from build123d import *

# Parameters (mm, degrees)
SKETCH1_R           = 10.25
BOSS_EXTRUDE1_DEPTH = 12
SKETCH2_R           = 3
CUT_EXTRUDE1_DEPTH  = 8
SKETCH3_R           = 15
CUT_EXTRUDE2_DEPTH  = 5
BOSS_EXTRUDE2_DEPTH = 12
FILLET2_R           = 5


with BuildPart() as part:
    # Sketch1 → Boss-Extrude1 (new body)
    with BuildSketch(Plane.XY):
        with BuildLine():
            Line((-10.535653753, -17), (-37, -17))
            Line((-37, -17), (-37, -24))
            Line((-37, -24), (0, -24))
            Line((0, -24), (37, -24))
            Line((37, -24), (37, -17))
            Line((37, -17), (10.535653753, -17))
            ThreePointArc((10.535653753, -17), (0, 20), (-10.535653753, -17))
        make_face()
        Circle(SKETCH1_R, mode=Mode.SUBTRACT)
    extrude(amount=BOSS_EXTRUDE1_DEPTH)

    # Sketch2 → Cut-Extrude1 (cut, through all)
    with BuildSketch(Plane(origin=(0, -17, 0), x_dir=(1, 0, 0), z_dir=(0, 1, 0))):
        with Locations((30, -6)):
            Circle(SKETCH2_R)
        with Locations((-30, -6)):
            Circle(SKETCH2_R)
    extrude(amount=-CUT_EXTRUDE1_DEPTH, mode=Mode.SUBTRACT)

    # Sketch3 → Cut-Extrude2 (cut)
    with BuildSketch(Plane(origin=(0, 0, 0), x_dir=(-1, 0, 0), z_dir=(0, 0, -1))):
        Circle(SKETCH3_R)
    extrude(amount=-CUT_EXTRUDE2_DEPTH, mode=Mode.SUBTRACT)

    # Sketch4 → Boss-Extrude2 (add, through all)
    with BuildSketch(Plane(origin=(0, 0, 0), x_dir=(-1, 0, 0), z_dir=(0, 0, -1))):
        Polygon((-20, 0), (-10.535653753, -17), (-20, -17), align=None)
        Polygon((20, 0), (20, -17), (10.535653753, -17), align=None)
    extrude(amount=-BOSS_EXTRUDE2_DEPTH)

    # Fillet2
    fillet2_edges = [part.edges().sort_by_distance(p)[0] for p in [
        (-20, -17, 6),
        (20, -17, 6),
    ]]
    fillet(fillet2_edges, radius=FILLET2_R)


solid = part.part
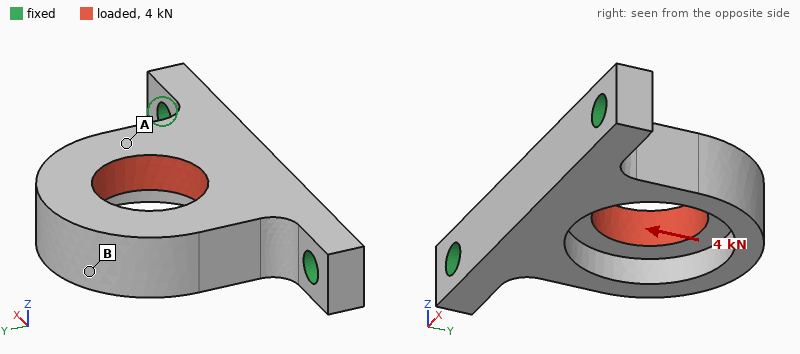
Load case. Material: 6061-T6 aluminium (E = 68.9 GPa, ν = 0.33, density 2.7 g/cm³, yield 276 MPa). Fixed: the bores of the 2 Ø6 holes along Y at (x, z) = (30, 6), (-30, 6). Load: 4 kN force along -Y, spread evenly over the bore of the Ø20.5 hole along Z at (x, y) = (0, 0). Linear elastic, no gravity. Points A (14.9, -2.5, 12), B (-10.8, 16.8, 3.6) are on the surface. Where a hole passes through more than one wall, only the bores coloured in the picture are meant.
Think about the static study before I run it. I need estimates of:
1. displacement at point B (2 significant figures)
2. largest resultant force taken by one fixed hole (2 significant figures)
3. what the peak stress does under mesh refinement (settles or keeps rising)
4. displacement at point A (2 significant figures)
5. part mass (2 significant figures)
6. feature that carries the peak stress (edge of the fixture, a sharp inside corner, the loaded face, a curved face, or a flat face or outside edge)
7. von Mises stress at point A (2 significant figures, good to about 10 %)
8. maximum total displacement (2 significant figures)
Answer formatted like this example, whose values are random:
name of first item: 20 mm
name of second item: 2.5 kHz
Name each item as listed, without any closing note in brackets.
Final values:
displacement at point B: 0.085 mm
largest resultant force taken by one fixed hole: 2.3 kN
what the peak stress does under mesh refinement: keeps rising
displacement at point A: 0.051 mm
part mass: 43 g
feature that carries the peak stress: edge of the fixture
von Mises stress at point A: 28 MPa
maximum total displacement: 0.10 mm
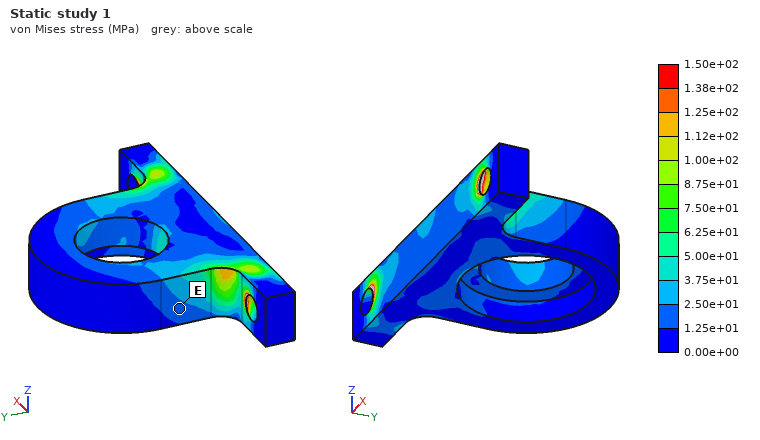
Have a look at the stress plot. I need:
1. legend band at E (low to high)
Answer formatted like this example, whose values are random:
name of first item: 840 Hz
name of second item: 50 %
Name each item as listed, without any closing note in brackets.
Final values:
legend band at E: 1.25e+01 to 2.50e+01 MPa
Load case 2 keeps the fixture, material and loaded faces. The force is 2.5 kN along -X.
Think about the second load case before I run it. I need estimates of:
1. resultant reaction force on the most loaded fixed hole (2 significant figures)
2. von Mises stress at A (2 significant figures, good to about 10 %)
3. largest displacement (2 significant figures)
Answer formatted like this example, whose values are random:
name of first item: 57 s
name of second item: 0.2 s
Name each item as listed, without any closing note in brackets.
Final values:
resultant reaction force on the most loaded fixed hole: 1.6 kN
von Mises stress at A: 23 MPa
largest displacement: 35 µm
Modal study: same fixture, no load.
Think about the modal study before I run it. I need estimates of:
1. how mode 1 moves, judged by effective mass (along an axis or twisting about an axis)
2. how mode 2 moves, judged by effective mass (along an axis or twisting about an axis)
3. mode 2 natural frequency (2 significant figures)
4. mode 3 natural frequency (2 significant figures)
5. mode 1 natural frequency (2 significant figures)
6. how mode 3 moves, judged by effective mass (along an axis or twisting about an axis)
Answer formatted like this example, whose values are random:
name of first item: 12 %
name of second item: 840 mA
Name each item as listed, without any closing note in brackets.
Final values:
how mode 1 moves, judged by effective mass: along Z
how mode 2 moves, judged by effective mass: along X
mode 2 natural frequency: 8600 Hz
mode 3 natural frequency: 10 kHz
mode 1 natural frequency: 2800 Hz
how mode 3 moves, judged by effective mass: along X
